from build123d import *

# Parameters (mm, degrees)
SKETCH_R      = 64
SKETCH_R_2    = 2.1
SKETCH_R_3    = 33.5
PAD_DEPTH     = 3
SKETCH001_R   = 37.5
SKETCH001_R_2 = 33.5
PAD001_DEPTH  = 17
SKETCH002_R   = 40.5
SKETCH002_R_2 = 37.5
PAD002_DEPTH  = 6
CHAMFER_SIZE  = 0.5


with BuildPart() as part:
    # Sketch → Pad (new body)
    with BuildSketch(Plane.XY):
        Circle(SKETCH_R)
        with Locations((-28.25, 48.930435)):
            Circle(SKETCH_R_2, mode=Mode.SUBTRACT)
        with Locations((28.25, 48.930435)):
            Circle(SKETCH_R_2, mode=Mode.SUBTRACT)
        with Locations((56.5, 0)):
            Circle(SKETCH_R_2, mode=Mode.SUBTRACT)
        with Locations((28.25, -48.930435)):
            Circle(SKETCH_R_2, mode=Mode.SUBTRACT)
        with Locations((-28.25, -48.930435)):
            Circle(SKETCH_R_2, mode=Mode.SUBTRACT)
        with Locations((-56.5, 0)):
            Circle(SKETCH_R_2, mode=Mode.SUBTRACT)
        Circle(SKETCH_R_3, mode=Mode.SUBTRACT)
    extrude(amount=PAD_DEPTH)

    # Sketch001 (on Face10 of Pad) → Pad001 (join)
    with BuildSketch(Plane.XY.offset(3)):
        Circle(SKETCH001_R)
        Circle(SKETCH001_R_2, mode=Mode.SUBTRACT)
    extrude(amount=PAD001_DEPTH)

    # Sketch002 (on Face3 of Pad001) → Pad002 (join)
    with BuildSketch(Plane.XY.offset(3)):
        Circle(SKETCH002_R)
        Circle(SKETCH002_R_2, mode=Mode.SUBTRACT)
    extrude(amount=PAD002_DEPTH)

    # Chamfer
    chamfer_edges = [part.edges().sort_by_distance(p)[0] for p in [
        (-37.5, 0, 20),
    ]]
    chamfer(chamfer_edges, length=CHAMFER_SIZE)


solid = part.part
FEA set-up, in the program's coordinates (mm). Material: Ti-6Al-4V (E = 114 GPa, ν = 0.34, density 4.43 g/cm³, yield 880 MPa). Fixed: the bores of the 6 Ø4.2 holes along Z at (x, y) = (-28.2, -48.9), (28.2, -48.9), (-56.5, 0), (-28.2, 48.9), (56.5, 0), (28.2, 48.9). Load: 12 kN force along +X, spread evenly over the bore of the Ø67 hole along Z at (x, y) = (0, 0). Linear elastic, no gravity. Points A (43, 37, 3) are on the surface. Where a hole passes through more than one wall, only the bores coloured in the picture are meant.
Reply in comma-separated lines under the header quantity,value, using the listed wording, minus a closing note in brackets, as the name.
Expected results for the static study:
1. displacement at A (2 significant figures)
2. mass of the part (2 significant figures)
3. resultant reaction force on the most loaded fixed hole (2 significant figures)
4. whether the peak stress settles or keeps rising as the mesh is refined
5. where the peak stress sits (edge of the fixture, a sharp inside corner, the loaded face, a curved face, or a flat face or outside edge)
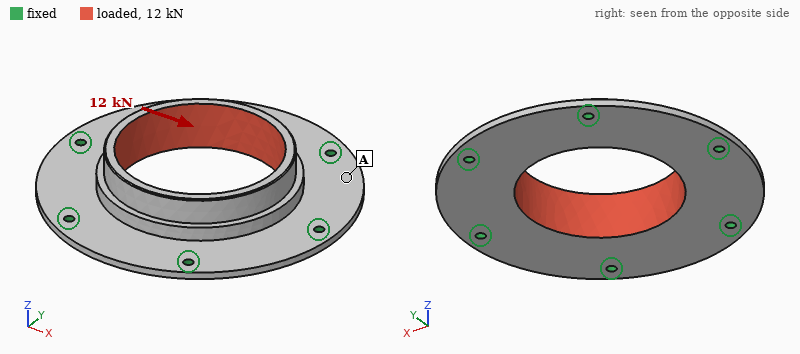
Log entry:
quantity,value
displacement at A,18 µm
mass of the part,210 g
resultant reaction force on the most loaded fixed hole,2.4 kN
whether the peak stress settles or keeps rising as the mesh is refined,keeps rising
where the peak stress sits,edge of the fixture
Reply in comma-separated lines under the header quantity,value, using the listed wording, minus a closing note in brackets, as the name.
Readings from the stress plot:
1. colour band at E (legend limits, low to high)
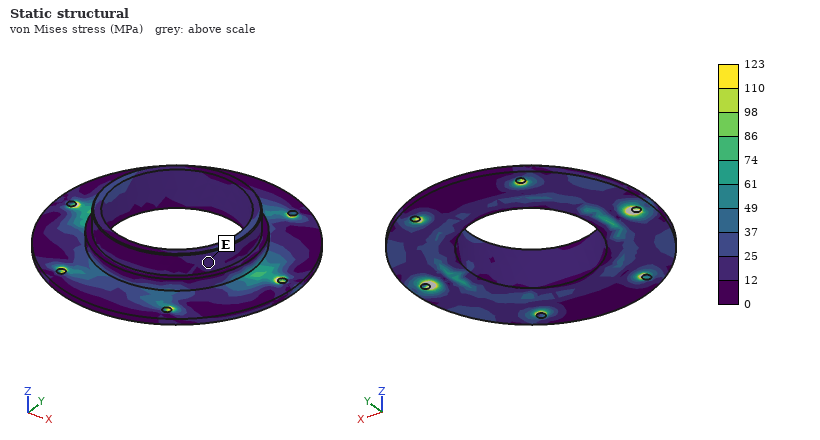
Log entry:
quantity,value
colour band at E,12 to 25 MPa
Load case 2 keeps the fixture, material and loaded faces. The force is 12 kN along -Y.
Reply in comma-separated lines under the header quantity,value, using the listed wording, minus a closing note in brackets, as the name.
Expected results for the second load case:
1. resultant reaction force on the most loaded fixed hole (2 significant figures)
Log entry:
quantity,value
resultant reaction force on the most loaded fixed hole,2.3 kN
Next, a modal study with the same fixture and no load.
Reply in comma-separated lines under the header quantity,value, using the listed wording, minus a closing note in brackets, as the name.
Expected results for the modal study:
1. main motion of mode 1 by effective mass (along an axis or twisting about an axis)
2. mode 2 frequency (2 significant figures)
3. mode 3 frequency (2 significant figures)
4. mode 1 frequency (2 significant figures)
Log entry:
quantity,value
main motion of mode 1 by effective mass,along Z
mode 2 frequency,4500 Hz
mode 3 frequency,4500 Hz
mode 1 frequency,3800 Hz
